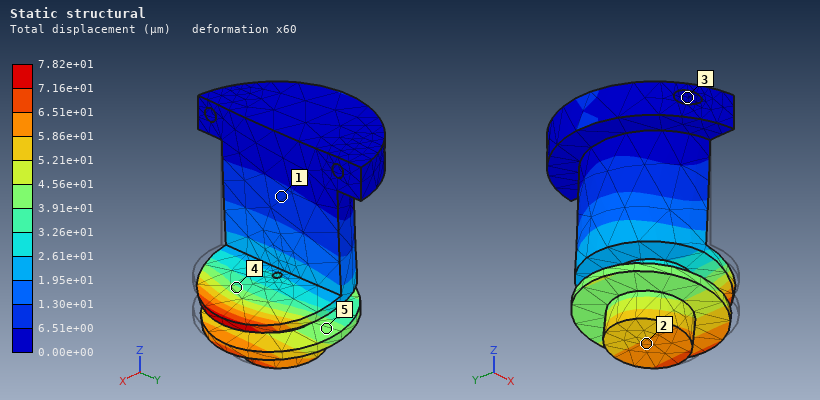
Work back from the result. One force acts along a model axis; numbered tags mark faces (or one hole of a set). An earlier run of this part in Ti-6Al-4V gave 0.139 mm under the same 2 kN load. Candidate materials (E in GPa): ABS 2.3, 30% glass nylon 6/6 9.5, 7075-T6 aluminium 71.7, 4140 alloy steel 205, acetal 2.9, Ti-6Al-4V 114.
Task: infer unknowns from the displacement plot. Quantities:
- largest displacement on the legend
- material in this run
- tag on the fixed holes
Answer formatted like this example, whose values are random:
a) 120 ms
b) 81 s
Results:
a) 7.82e+01 µm
b) 4140 alloy steel
c) 3
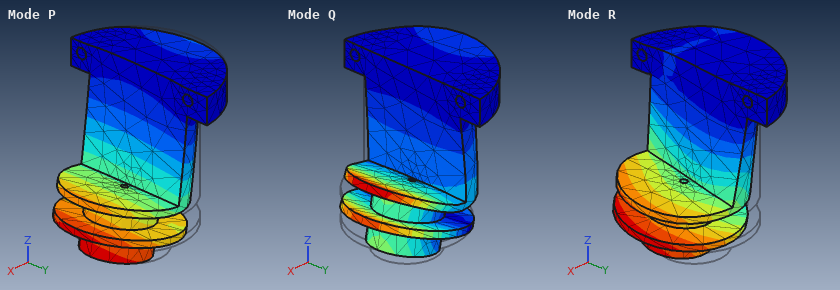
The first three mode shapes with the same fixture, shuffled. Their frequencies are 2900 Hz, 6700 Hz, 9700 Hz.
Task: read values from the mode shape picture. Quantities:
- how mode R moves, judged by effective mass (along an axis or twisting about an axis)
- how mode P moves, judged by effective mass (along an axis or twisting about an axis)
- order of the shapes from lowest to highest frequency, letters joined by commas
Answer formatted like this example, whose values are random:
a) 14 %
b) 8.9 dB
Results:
a) along Y
b) along X
c) P, R, Q
